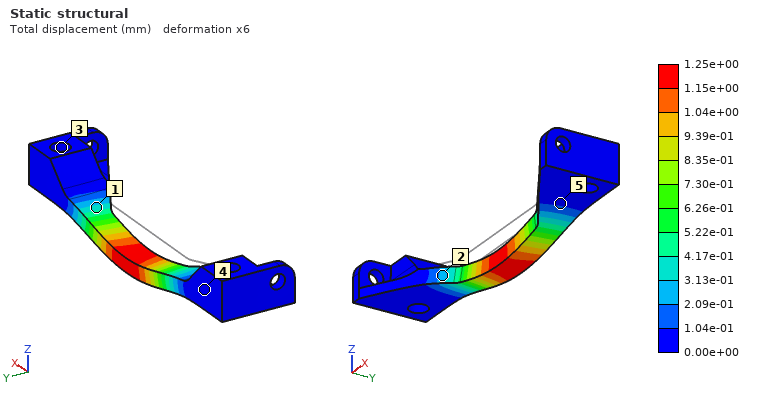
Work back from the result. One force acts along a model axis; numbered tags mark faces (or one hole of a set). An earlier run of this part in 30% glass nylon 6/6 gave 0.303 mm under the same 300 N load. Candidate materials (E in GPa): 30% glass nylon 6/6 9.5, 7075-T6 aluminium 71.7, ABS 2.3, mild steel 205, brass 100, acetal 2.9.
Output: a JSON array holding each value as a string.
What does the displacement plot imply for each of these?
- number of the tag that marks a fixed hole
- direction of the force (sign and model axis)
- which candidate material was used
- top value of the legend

["3", "-Z", "ABS", "1.25e+00 mm"]
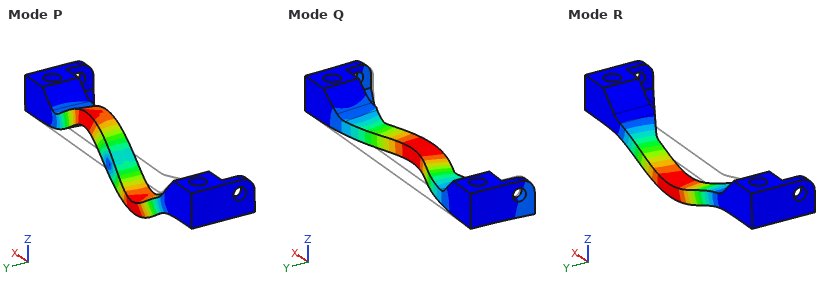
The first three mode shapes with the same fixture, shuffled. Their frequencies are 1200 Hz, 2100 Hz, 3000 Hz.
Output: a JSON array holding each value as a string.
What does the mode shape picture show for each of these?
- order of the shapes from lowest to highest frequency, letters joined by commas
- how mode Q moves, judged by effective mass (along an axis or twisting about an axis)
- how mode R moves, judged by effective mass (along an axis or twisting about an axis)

["R, Q, P", "along Y", "along Z"]
